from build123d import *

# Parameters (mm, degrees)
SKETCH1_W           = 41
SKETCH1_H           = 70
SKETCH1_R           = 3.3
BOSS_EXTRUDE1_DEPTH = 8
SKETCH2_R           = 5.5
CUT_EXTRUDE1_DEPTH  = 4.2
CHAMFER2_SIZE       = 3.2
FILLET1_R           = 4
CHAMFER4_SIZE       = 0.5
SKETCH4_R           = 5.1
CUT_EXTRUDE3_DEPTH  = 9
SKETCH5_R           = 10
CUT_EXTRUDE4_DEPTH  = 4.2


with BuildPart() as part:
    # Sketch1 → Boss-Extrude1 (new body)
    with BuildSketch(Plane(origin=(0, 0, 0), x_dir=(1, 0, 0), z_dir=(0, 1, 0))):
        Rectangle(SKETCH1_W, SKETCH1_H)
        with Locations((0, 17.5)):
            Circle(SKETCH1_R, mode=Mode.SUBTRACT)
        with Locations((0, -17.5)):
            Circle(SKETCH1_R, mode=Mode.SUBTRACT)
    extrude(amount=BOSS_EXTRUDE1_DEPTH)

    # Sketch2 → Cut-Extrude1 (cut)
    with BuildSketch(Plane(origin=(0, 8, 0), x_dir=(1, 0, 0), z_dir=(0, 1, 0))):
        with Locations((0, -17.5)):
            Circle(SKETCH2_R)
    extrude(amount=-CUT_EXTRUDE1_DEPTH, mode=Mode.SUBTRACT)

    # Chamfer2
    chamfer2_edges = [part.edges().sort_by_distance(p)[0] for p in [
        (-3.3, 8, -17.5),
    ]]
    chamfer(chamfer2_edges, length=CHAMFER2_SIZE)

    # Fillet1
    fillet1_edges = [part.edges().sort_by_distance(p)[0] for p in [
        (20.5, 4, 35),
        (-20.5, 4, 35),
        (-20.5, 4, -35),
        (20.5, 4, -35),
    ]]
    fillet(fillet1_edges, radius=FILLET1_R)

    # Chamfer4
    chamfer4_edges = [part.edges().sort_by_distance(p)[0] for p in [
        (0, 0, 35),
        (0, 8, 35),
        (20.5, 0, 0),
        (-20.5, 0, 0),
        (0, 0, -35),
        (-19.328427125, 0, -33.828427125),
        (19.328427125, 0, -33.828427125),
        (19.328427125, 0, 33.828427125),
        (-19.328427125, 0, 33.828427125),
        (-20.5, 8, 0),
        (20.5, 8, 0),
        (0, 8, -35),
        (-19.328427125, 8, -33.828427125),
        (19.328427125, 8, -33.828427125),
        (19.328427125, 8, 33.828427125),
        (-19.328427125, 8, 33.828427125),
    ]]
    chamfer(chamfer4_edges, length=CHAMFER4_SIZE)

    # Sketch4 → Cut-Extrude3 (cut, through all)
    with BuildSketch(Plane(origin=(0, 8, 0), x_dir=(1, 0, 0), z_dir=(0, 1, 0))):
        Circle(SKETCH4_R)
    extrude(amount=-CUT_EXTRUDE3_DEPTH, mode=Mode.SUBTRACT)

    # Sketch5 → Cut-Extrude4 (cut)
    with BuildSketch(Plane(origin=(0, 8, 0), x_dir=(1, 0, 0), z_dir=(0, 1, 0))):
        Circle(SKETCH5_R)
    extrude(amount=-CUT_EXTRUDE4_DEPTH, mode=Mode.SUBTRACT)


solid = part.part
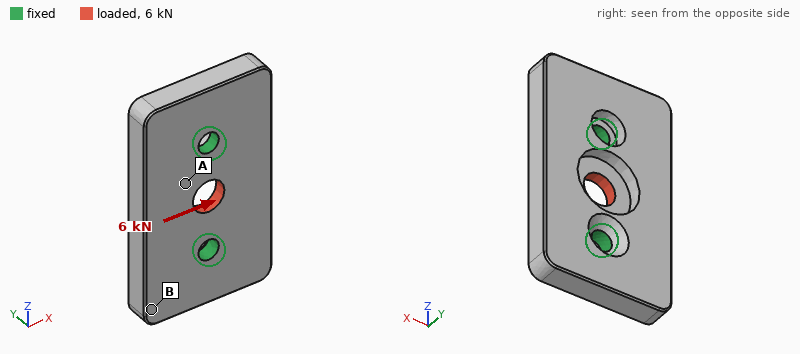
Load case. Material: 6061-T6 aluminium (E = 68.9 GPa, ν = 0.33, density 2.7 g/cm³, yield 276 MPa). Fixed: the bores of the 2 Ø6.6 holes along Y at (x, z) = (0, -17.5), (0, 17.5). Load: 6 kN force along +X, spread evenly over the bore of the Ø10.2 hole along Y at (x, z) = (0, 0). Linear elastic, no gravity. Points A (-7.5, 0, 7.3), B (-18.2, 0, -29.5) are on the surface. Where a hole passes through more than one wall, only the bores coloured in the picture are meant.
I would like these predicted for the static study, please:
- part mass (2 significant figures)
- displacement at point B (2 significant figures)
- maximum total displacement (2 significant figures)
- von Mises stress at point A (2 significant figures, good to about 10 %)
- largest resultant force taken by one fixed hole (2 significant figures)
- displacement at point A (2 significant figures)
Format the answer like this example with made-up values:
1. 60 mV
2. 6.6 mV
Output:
1. 55 g
2. 4.1 µm
3. 15 µm
4. 38 MPa
5. 3.0 kN
6. 8.7 µm
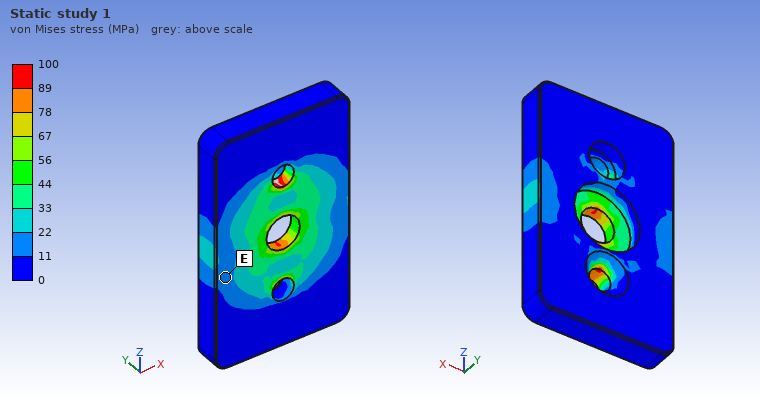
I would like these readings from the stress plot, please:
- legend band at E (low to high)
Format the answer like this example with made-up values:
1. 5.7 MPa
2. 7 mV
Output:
1. 11 to 22 MPa
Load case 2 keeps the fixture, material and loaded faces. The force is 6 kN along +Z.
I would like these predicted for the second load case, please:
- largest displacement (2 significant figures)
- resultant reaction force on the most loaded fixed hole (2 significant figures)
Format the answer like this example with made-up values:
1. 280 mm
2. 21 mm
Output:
1. 9.3 µm
2. 3.2 kN
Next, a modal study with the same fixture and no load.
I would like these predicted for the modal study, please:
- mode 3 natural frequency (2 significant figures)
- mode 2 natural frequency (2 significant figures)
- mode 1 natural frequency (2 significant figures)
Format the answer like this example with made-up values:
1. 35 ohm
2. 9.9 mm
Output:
1. 11 kHz
2. 10000 Hz
3. 6800 Hz
